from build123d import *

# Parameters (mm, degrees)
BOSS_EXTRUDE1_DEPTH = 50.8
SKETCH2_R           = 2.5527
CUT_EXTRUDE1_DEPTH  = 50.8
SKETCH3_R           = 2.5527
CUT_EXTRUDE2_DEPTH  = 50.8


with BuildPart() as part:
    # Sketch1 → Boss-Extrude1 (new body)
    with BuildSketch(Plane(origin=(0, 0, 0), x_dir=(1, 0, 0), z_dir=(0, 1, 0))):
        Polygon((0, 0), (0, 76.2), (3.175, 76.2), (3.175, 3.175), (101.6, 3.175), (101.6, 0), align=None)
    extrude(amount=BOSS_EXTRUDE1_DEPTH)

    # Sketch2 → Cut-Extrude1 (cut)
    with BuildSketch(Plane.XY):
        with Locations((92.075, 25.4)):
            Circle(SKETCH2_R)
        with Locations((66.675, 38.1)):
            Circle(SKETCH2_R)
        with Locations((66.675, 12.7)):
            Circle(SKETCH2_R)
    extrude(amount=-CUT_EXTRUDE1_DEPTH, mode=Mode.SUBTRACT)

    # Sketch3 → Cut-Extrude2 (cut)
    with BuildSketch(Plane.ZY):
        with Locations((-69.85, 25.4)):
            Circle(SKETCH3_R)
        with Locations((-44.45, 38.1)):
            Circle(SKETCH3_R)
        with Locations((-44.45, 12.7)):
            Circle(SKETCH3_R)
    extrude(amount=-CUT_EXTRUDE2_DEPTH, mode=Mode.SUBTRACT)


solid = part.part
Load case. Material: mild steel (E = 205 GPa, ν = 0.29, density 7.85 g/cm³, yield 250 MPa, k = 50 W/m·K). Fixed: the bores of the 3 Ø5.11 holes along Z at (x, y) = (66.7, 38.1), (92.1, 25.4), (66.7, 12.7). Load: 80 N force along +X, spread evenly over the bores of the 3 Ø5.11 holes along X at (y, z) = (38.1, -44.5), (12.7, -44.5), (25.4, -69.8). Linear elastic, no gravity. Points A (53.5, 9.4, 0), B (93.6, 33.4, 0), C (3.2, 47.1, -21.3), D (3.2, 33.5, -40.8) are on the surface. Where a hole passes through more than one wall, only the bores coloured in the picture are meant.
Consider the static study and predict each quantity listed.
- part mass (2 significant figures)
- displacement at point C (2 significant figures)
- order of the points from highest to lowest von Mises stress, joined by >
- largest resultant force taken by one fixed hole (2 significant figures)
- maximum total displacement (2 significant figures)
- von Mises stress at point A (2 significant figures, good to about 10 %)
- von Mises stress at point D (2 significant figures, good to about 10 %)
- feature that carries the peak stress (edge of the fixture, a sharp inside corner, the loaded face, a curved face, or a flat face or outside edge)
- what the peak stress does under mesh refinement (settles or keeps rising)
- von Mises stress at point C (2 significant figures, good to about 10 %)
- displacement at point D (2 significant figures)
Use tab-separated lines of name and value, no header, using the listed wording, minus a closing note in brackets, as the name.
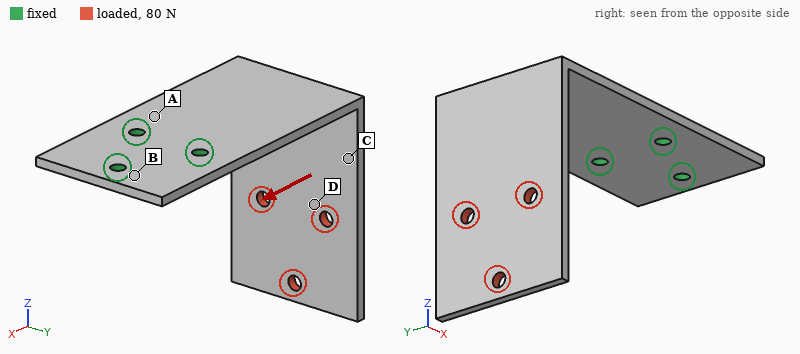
part mass	220 g
displacement at point C	0.34 mm
order of the points from highest to lowest von Mises stress, joined by >	A > C > D > B
largest resultant force taken by one fixed hole	38 N
maximum total displacement	0.94 mm
von Mises stress at point A	45 MPa
von Mises stress at point D	13 MPa
feature that carries the peak stress	edge of the fixture
what the peak stress does under mesh refinement	keeps rising
von Mises stress at point C	29 MPa
displacement at point D	0.52 mm
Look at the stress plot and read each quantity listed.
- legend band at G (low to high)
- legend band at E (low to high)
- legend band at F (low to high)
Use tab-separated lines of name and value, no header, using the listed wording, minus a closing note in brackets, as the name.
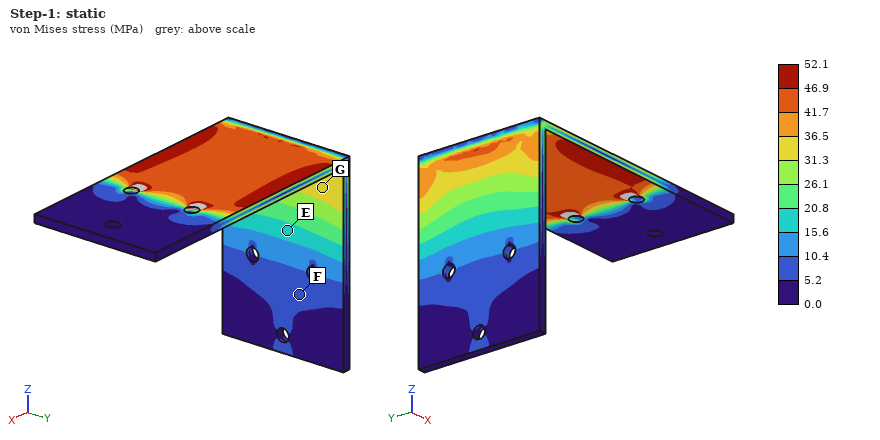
legend band at G	31.3 to 36.5 MPa
legend band at E	15.6 to 20.8 MPa
legend band at F	5.2 to 10.4 MPa
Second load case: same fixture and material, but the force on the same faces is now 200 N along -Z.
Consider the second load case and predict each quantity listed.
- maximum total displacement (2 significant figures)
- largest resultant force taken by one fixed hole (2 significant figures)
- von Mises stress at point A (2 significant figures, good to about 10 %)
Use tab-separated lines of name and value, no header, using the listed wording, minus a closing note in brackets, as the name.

maximum total displacement	1.3 mm
largest resultant force taken by one fixed hole	130 N
von Mises stress at point A	110 MPa
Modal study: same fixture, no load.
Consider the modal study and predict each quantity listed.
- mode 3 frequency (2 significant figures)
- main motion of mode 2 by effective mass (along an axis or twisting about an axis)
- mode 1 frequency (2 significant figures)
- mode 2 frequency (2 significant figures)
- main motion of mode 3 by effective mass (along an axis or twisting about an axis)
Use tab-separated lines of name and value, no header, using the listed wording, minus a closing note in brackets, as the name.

mode 3 frequency	510 Hz
main motion of mode 2 by effective mass	along Y
mode 1 frequency	190 Hz
mode 2 frequency	330 Hz
main motion of mode 3 by effective mass	along Z
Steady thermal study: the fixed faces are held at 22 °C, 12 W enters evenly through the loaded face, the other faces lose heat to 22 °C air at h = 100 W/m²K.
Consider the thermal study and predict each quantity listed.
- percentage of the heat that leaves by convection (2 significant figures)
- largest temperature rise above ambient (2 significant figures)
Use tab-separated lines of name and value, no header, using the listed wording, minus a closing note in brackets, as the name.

percentage of the heat that leaves by convection	98 %
largest temperature rise above ambient	27 K
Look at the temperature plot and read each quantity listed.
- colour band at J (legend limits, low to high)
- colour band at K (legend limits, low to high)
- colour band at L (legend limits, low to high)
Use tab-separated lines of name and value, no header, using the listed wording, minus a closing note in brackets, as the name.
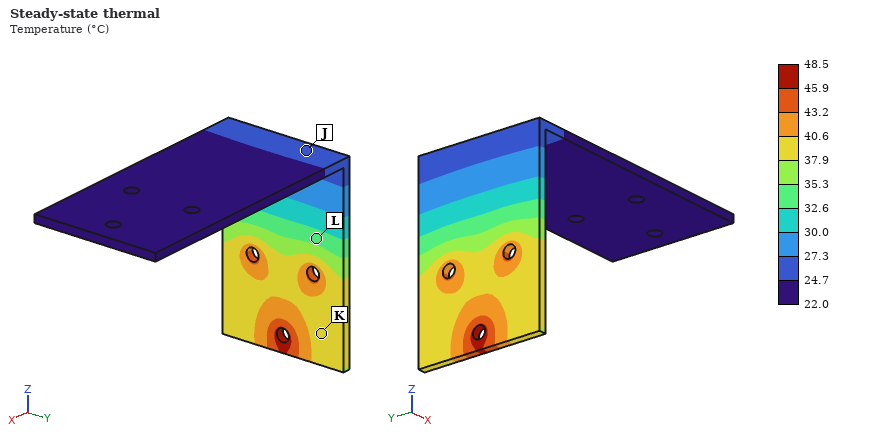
colour band at J	24.7 to 27.3 °C
colour band at K	37.9 to 40.6 °C
colour band at L	32.6 to 35.3 °C
